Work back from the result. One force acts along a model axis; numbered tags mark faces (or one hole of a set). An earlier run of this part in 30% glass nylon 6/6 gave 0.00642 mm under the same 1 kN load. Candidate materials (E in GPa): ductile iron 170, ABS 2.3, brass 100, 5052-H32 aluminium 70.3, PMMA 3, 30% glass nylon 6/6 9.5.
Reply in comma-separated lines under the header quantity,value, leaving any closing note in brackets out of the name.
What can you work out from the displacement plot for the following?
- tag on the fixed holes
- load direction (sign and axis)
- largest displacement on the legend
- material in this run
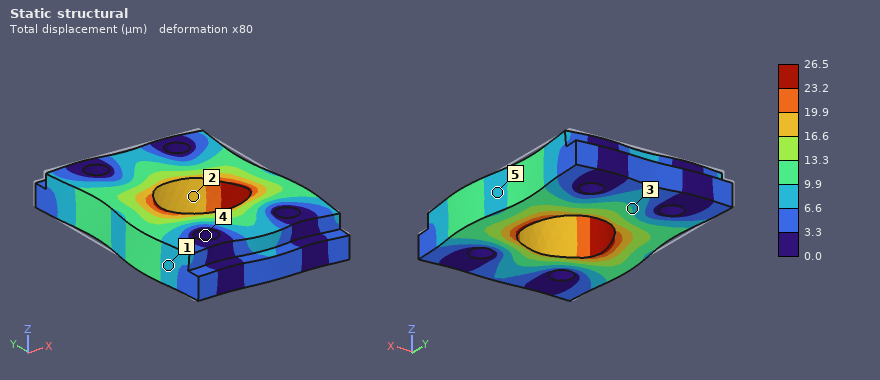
quantity,value
tag on the fixed holes,4
load direction,-Y
largest displacement on the legend,26.5 µm
material in this run,ABS
